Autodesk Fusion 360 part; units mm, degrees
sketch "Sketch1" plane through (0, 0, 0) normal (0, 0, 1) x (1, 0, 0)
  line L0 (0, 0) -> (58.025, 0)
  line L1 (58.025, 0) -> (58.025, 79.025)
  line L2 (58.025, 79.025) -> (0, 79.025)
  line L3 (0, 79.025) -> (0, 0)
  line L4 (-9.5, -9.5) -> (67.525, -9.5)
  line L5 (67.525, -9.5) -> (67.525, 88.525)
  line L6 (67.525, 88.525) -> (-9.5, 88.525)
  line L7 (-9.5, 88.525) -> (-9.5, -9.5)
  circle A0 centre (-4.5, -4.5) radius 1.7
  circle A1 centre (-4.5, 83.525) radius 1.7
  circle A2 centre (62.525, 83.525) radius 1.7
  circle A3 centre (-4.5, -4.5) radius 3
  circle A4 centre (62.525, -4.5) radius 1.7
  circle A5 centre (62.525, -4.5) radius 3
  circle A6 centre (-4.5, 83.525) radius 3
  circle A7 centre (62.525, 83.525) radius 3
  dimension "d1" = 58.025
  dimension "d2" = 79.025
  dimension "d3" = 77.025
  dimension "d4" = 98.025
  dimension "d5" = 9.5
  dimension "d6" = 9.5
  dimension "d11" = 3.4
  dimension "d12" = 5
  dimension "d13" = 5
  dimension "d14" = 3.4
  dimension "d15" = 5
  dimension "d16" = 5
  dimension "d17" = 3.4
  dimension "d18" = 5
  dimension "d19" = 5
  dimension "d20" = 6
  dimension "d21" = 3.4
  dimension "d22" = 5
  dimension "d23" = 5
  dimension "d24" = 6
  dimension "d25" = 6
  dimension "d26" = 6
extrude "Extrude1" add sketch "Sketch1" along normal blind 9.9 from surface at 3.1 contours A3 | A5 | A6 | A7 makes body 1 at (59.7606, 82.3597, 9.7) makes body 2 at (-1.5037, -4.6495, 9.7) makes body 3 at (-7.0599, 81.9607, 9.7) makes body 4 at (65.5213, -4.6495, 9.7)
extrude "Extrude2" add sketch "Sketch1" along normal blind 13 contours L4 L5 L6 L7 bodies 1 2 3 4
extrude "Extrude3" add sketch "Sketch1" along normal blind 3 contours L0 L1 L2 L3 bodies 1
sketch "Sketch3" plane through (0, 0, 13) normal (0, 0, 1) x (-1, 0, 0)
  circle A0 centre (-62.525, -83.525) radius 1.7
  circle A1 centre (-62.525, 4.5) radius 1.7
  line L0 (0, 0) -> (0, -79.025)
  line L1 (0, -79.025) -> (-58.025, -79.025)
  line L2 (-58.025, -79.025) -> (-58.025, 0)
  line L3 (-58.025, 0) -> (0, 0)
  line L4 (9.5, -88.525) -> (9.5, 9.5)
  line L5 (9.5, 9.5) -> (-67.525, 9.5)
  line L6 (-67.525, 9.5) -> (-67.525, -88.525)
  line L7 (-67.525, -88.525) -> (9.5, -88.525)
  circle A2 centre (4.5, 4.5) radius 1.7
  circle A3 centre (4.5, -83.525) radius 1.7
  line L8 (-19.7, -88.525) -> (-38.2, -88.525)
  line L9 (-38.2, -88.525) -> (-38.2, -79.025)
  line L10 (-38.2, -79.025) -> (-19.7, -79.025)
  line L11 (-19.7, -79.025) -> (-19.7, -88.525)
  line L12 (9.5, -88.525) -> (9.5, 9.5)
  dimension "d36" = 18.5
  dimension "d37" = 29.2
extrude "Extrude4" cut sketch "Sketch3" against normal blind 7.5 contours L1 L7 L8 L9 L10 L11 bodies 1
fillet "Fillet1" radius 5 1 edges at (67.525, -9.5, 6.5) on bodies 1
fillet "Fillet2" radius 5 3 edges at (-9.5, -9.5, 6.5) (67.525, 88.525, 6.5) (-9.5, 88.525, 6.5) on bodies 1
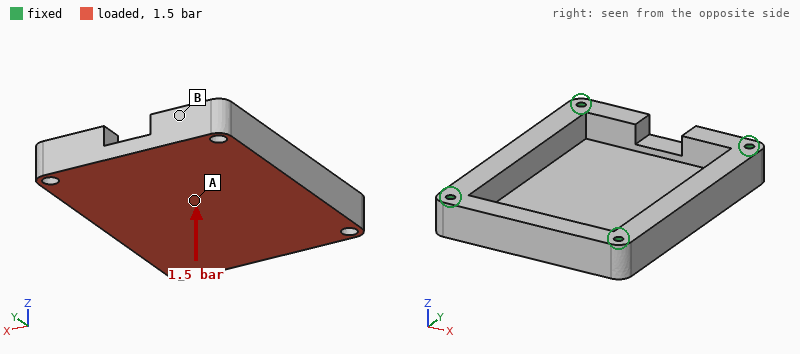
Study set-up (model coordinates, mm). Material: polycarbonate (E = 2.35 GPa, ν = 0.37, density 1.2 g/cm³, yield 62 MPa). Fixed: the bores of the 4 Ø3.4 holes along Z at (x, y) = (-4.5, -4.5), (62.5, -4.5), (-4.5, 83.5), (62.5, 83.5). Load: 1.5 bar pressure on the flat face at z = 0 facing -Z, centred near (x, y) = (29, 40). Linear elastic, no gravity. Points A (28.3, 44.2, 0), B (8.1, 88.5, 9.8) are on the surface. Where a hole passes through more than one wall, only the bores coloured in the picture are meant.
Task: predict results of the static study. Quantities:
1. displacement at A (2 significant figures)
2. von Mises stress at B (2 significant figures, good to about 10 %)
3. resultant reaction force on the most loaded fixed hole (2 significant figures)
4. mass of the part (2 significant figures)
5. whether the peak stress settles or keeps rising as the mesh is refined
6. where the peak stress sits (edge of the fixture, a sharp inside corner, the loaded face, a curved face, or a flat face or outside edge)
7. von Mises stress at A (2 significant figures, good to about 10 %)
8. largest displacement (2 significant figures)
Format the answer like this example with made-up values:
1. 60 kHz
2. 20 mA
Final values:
1. 1.1 mm
2. 2.3 MPa
3. 420 N
4. 60 g
5. keeps rising
6. edge of the fixture
7. 14 MPa
8. 1.1 mm
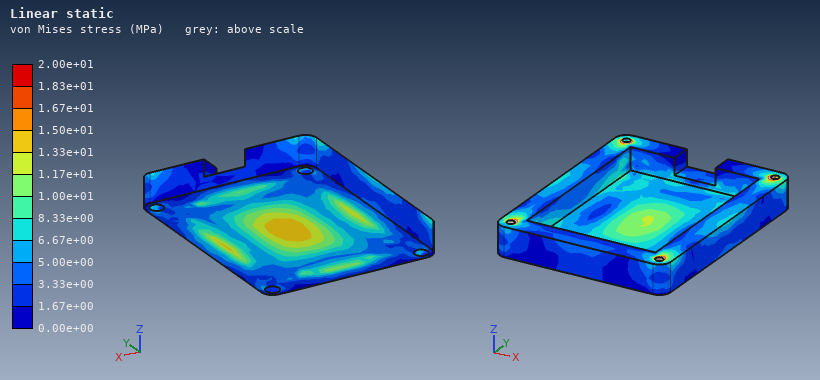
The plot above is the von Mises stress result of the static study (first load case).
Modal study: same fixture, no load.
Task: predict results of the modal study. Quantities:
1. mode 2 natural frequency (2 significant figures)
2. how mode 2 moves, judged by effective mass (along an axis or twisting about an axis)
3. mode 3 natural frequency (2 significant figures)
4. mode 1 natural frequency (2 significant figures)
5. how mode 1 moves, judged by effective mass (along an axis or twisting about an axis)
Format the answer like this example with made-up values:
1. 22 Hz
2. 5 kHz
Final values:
1. 1800 Hz
2. twisting about Y
3. 2100 Hz
4. 1200 Hz
5. along Z
